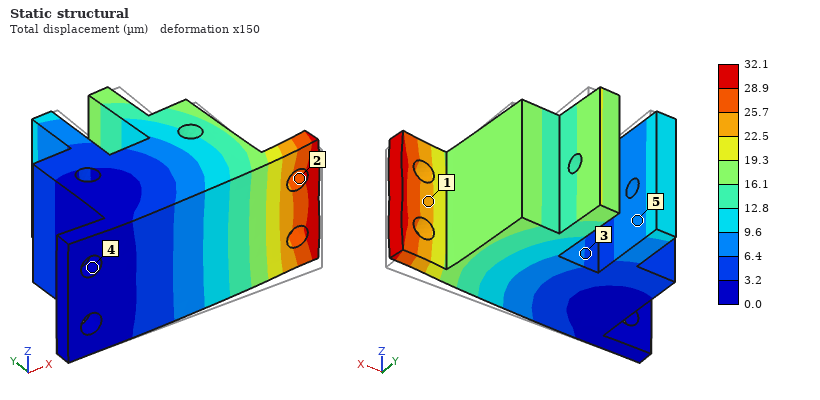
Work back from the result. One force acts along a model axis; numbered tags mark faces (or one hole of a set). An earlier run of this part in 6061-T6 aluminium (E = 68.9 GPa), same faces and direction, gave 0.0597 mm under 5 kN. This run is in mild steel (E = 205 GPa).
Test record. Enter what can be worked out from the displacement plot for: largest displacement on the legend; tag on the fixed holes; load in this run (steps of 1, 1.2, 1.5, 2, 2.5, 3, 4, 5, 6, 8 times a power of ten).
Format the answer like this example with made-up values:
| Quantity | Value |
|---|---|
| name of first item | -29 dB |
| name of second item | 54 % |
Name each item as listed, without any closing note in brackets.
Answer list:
| Quantity | Value |
|---|---|
| largest displacement on the legend | 32.1 µm |
| tag on the fixed holes | 4 |
| load in this run | 8 kN |
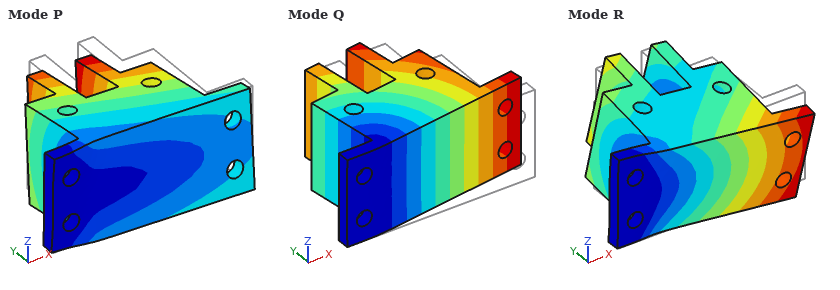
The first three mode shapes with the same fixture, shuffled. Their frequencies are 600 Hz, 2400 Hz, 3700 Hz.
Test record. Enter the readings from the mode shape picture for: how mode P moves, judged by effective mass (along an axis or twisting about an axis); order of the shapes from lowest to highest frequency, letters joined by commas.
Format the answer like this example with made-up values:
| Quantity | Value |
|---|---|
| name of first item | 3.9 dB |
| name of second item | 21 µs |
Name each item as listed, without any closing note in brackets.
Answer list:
| Quantity | Value |
|---|---|
| how mode P moves, judged by effective mass | along Z |
| order of the shapes from lowest to highest frequency, letters joined by commas | Q, P, R |
